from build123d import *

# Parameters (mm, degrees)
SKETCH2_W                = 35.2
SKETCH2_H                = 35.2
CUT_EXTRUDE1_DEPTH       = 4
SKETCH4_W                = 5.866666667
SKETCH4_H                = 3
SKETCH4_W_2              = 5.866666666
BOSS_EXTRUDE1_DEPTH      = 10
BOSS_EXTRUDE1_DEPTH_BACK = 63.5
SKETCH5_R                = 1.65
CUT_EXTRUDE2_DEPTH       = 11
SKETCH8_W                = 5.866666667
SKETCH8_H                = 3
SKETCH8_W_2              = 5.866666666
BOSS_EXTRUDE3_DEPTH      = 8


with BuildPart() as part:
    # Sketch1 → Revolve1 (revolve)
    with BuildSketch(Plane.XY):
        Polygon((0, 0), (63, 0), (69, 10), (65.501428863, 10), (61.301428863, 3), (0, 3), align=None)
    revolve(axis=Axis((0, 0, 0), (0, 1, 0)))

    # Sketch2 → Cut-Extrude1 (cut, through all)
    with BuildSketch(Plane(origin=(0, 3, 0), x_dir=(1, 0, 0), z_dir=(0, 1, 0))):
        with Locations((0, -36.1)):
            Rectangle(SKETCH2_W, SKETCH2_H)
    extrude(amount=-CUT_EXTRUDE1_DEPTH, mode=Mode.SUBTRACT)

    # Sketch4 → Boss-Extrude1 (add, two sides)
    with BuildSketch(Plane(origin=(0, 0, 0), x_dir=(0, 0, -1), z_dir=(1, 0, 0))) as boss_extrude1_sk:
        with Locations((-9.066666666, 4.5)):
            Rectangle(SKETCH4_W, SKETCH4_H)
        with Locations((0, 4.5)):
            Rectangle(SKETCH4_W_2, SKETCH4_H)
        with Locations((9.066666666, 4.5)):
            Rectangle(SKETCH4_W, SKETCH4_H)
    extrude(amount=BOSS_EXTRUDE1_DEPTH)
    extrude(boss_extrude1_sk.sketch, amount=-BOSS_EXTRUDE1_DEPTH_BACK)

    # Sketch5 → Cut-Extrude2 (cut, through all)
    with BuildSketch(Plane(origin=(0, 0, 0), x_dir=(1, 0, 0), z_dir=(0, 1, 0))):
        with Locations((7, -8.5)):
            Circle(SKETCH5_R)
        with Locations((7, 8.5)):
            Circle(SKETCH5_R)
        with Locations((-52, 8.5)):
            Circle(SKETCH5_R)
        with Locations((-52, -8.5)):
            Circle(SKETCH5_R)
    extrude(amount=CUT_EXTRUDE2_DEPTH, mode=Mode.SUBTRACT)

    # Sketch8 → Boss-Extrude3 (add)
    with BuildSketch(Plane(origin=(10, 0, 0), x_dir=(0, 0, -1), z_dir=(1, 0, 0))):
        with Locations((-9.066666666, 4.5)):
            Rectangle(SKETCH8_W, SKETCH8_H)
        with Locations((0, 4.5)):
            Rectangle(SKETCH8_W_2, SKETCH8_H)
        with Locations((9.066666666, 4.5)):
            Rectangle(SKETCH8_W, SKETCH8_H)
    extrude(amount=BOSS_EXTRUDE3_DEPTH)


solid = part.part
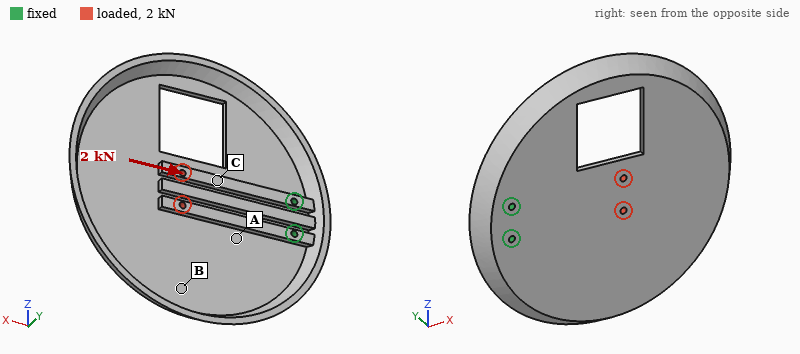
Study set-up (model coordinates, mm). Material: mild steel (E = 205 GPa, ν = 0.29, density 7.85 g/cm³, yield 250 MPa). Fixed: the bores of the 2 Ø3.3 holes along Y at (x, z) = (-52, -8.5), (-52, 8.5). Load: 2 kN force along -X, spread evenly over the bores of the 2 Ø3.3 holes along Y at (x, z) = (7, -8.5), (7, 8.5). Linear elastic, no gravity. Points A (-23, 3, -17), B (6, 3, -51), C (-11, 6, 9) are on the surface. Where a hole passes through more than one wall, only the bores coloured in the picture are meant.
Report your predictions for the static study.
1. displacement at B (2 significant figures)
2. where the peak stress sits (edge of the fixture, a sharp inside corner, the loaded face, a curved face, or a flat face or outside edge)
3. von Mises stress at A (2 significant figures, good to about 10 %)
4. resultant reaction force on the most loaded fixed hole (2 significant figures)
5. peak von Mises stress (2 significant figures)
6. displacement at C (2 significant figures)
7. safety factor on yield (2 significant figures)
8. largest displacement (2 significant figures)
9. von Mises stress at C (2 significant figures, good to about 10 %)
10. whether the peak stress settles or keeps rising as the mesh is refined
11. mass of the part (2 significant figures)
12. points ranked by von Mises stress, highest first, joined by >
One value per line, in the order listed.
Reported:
13 µm
the loaded face
9.1 MPa
1.0 kN
47 MPa
7.3 µm
5.3
41 µm
19 MPa
settles
380 g
C > A > B
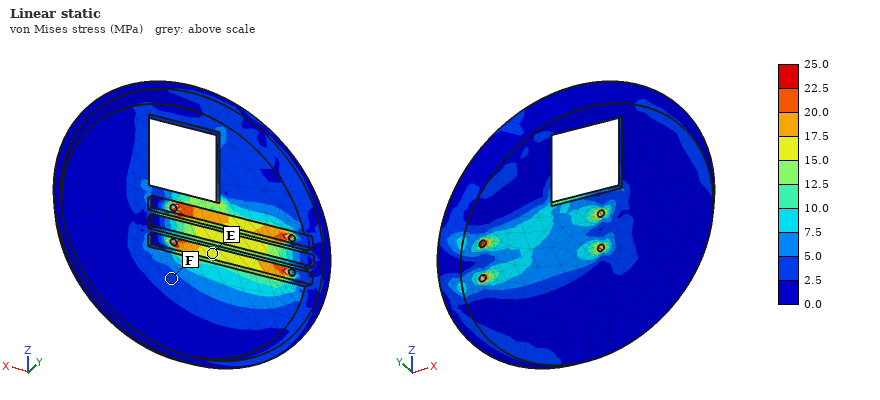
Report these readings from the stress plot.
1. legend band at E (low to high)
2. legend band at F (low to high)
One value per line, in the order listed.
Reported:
15.0 to 17.5 MPa
2.5 to 5.0 MPa
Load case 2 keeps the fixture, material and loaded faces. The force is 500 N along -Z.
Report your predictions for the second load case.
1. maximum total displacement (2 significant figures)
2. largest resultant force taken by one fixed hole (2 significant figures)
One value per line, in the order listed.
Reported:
29 µm
1.5 kN
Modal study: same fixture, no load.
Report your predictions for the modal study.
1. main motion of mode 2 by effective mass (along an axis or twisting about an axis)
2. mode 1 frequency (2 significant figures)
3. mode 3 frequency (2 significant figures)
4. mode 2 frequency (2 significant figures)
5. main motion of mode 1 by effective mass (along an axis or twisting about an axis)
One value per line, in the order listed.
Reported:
twisting about X
300 Hz
1200 Hz
580 Hz
along Y
